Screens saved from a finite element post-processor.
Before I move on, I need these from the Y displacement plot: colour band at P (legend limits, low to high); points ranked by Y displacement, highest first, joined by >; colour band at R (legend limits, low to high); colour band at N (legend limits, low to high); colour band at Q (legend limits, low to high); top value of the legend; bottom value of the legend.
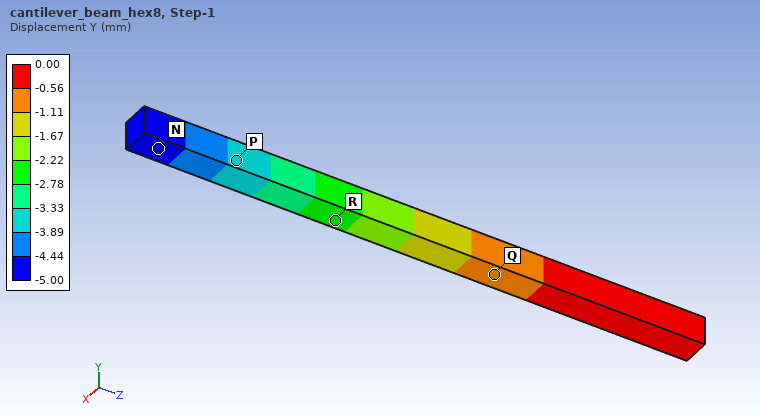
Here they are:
-3.89 to -3.33 mm
Q > R > P > N
-2.78 to -2.22 mm
-5.00 to -4.44 mm
-1.11 to -0.56 mm
0.00 mm
-5.00 mm
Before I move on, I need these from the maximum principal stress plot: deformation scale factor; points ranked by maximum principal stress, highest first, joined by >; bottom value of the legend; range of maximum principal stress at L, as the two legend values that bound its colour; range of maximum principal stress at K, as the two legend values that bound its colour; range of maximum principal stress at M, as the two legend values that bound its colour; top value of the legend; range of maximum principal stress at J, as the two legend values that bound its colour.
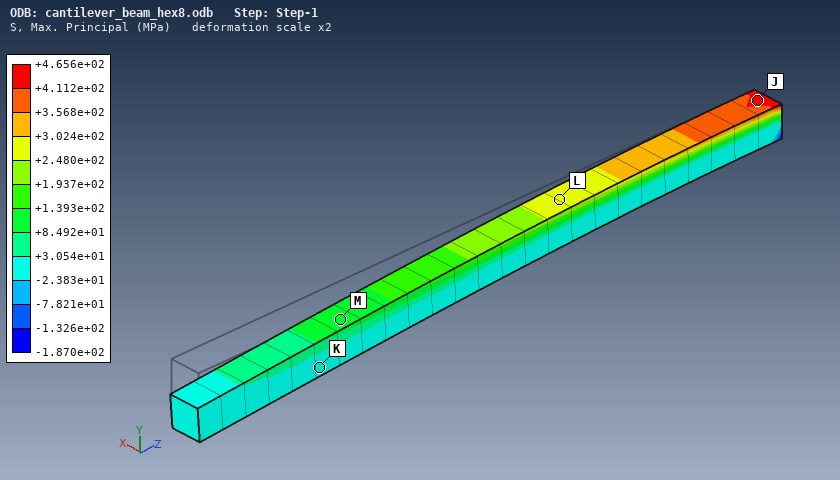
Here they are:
2
J > L > M > K
-1.870e+02 MPa
+2.480e+02 to +3.024e+02 MPa
-2.383e+01 to +3.054e+01 MPa
+8.492e+01 to +1.393e+02 MPa
+4.656e+02 MPa
+4.112e+02 to +4.656e+02 MPa
